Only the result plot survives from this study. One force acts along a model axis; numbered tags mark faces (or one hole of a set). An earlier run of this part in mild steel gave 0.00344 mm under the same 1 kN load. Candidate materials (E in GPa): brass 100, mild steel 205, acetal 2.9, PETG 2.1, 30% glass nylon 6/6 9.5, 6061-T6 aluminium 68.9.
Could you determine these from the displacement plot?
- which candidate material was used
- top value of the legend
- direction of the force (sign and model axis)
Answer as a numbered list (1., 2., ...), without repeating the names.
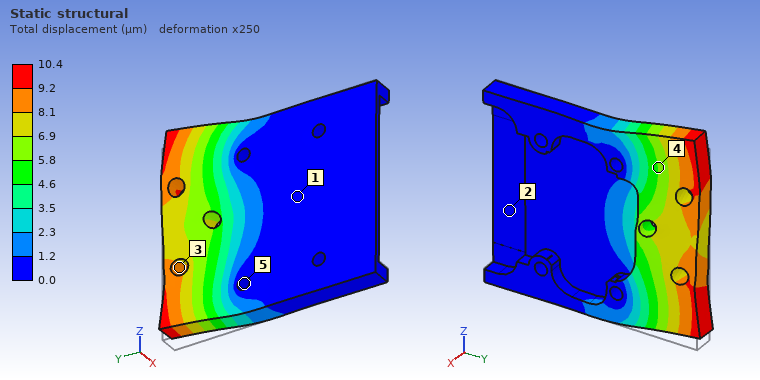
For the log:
1. 6061-T6 aluminium
2. 10.4 µm
3. +Z
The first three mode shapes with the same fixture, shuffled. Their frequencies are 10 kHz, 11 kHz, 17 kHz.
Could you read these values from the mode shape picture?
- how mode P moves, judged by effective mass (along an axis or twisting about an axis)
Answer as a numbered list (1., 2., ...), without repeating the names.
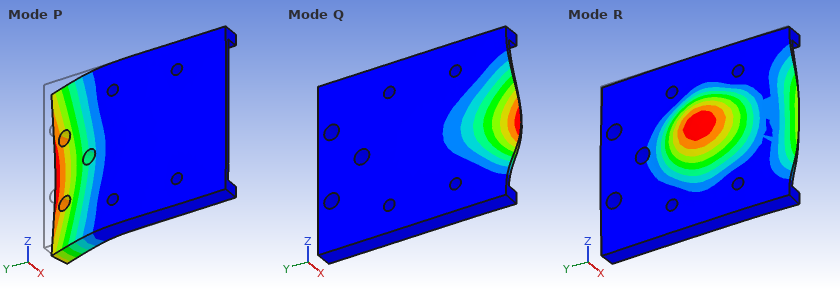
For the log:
1. along X
